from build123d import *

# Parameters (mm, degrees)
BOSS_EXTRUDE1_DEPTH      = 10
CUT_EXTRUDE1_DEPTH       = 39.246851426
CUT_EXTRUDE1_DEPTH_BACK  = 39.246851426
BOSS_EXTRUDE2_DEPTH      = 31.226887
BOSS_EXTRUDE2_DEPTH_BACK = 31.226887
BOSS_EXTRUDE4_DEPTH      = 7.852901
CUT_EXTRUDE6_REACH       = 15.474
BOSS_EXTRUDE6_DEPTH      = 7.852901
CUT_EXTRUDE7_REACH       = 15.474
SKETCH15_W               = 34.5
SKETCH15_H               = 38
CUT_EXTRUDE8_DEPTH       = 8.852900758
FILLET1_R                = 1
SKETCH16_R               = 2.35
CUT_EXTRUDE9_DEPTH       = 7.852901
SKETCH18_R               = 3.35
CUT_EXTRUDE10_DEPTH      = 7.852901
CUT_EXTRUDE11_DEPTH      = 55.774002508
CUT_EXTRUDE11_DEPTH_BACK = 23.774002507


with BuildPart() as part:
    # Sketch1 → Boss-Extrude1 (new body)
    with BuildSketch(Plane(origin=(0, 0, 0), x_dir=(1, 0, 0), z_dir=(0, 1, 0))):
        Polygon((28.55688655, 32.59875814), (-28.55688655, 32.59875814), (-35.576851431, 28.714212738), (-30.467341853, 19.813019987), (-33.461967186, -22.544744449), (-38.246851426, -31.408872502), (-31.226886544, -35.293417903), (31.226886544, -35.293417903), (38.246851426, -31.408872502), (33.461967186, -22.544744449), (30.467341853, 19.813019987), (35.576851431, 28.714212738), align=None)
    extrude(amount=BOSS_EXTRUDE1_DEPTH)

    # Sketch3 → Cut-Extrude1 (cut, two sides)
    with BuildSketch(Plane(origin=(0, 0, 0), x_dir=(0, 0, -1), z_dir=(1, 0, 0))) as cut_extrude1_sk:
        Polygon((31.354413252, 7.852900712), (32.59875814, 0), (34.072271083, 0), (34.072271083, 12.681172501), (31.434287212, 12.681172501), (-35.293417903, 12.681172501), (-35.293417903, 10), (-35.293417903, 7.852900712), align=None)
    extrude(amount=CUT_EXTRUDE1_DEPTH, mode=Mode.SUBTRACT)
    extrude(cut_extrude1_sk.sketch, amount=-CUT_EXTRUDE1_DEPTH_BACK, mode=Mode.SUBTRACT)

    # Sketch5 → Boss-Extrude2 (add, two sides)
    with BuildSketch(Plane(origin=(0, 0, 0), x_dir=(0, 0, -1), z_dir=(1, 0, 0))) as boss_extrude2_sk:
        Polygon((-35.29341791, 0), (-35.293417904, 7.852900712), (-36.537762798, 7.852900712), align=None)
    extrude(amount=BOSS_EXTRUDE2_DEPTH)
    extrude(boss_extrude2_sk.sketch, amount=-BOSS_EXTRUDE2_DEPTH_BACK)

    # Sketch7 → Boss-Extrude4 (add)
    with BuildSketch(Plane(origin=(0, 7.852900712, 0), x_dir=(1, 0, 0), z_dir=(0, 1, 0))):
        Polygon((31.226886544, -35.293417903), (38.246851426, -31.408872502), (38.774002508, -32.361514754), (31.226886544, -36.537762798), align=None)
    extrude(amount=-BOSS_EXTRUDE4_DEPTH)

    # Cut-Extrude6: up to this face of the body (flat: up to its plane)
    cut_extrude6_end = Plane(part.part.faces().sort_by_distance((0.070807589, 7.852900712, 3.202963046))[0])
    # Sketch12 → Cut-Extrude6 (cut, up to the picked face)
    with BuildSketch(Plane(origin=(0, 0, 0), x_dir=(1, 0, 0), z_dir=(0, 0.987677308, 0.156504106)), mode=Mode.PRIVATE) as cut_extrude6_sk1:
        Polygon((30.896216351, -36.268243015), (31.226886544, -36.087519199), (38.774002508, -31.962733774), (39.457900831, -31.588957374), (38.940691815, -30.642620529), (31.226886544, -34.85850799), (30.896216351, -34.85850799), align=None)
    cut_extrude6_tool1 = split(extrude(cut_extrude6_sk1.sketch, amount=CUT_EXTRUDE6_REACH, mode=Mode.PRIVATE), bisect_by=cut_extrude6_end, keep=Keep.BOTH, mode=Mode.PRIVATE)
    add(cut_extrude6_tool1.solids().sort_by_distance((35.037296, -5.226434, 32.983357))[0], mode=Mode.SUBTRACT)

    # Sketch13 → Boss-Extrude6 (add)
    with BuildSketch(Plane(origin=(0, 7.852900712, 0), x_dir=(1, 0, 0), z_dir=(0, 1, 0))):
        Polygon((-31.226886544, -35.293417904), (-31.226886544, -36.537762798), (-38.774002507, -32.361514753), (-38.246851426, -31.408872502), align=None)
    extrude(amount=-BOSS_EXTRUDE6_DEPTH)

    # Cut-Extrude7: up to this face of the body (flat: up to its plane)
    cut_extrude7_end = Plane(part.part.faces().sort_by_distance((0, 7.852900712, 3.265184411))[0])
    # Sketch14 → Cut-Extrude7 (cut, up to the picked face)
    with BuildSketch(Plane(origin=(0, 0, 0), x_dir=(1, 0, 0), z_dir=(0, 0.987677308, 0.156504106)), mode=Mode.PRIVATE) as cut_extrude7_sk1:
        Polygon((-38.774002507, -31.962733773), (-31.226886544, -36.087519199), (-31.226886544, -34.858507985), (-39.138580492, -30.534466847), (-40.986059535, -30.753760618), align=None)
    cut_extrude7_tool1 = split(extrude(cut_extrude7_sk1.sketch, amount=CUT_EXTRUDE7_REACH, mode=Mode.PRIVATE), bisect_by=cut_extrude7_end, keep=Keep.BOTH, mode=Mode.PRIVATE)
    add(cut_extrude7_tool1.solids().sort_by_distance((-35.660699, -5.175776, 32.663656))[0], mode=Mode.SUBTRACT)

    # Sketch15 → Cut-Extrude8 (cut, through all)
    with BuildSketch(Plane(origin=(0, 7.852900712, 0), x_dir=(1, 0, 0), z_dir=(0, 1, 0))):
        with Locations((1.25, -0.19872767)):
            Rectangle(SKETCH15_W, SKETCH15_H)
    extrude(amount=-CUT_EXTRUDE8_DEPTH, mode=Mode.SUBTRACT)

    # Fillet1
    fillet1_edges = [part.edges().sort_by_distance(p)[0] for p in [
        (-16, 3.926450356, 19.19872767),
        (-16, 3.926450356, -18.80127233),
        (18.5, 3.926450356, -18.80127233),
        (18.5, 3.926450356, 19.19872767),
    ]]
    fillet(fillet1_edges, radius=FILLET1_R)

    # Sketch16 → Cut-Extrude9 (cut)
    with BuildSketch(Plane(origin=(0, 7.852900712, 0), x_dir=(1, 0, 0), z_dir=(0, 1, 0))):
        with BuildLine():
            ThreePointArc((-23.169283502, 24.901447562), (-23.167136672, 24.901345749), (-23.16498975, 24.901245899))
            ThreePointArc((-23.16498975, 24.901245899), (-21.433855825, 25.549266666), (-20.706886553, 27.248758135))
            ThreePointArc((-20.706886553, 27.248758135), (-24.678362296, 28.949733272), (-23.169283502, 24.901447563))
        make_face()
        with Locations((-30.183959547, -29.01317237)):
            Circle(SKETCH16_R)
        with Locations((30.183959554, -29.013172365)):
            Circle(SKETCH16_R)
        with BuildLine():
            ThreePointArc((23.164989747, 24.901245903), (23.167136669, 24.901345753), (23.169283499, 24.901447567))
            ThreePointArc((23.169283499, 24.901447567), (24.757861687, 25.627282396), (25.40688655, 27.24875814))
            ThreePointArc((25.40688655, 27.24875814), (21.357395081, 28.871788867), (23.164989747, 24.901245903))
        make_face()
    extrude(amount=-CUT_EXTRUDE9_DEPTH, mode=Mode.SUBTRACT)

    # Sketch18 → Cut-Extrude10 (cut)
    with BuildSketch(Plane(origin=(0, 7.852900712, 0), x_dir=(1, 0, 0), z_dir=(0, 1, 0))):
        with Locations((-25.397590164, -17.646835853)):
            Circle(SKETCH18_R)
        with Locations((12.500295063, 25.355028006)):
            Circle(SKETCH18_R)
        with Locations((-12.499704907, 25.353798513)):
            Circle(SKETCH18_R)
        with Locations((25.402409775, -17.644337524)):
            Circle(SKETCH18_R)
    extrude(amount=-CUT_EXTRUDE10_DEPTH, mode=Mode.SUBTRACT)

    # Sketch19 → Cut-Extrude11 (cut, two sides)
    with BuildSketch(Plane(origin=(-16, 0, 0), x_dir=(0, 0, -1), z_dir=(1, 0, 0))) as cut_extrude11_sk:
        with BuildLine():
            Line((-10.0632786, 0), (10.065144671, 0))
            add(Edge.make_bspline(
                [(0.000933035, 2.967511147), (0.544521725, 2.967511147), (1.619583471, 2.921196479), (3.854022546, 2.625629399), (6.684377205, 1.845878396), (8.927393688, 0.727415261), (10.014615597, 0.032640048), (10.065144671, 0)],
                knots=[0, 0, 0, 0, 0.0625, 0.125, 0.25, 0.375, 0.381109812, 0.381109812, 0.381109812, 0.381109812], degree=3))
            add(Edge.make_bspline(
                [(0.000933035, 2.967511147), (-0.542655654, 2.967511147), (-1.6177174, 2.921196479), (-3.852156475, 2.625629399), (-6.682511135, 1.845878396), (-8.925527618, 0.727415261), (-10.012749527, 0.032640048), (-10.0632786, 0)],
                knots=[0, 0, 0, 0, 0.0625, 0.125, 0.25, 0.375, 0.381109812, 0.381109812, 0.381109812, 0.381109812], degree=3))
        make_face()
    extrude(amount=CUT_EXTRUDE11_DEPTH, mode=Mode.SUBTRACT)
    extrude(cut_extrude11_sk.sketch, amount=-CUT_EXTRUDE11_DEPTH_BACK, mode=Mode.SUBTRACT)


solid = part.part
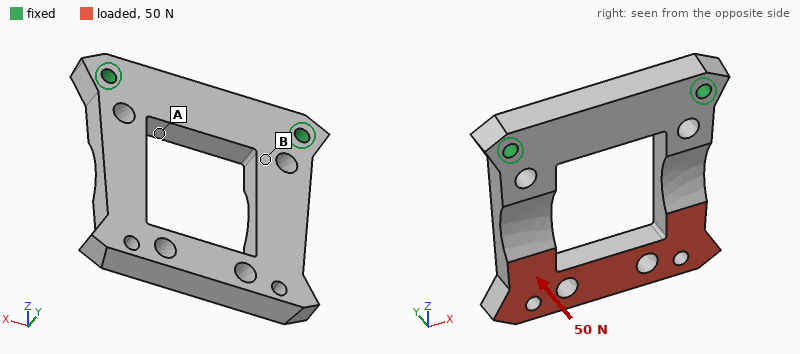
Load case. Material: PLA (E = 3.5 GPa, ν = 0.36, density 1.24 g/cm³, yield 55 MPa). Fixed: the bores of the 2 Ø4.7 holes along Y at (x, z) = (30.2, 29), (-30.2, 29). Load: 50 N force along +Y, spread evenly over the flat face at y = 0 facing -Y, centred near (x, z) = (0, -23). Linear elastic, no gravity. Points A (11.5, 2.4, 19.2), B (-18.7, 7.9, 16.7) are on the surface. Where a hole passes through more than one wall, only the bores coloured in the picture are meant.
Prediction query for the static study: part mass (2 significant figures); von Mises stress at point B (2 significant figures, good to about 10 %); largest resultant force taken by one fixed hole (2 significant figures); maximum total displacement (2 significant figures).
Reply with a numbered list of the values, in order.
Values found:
1. 27 g
2. 7.8 MPa
3. 26 N
4. 1.2 mm
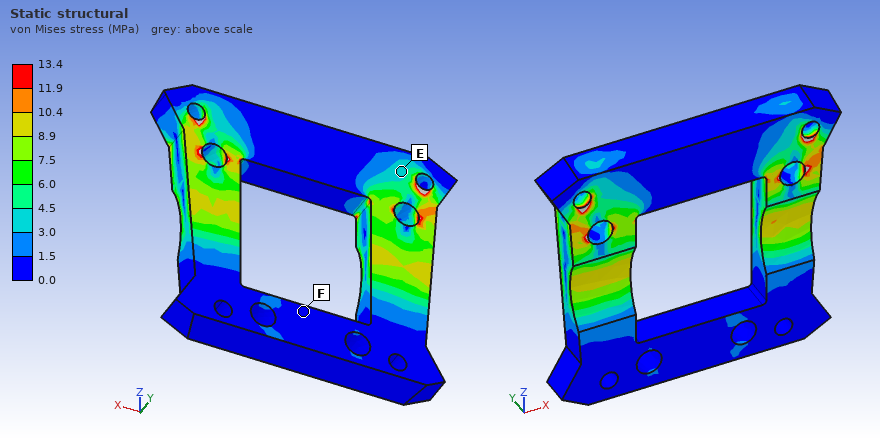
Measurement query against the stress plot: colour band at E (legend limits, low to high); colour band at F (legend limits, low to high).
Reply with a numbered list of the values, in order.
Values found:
1. 3.0 to 4.5 MPa
2. 0.0 to 1.5 MPa
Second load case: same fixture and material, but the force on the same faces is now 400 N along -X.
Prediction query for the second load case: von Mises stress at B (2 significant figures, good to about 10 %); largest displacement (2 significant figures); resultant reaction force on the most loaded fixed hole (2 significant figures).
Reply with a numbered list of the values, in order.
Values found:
1. 5.2 MPa
2. 0.84 mm
3. 360 N
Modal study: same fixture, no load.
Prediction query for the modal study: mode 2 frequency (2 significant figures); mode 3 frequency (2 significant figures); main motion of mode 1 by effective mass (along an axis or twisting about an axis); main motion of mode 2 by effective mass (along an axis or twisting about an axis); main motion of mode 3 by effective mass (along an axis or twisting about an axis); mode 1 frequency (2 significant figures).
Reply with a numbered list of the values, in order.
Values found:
1. 860 Hz
2. 1400 Hz
3. along Y
4. twisting about Z
5. along X
6. 360 Hz
